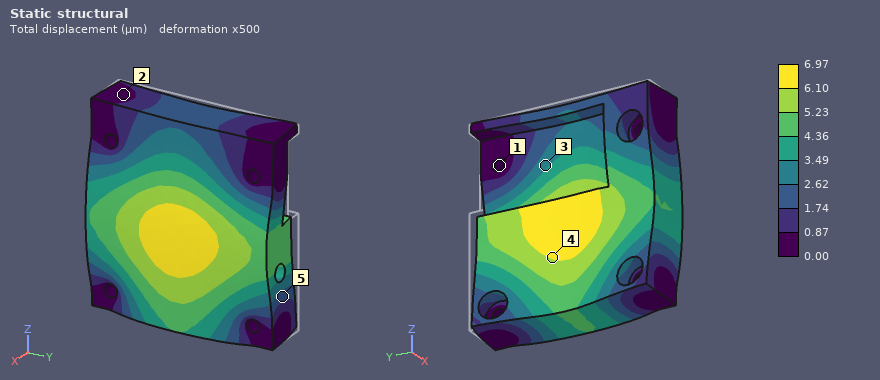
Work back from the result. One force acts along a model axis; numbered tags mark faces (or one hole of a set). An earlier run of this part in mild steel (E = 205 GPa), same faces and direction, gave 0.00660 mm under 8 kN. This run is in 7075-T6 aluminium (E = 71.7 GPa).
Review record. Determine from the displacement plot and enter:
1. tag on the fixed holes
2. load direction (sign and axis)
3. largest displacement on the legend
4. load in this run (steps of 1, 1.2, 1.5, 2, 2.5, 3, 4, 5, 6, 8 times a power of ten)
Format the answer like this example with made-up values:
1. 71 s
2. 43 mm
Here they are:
1. 1
2. +X
3. 6.97 µm
4. 3 kN
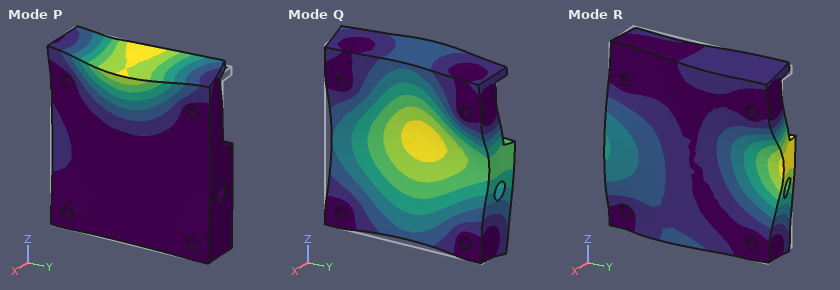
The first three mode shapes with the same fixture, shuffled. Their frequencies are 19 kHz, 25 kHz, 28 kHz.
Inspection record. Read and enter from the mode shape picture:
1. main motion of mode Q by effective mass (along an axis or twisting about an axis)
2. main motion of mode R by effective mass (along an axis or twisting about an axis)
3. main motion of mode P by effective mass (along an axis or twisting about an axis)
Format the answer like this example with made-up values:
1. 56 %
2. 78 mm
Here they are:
1. along X
2. twisting about Z
3. twisting about Y
